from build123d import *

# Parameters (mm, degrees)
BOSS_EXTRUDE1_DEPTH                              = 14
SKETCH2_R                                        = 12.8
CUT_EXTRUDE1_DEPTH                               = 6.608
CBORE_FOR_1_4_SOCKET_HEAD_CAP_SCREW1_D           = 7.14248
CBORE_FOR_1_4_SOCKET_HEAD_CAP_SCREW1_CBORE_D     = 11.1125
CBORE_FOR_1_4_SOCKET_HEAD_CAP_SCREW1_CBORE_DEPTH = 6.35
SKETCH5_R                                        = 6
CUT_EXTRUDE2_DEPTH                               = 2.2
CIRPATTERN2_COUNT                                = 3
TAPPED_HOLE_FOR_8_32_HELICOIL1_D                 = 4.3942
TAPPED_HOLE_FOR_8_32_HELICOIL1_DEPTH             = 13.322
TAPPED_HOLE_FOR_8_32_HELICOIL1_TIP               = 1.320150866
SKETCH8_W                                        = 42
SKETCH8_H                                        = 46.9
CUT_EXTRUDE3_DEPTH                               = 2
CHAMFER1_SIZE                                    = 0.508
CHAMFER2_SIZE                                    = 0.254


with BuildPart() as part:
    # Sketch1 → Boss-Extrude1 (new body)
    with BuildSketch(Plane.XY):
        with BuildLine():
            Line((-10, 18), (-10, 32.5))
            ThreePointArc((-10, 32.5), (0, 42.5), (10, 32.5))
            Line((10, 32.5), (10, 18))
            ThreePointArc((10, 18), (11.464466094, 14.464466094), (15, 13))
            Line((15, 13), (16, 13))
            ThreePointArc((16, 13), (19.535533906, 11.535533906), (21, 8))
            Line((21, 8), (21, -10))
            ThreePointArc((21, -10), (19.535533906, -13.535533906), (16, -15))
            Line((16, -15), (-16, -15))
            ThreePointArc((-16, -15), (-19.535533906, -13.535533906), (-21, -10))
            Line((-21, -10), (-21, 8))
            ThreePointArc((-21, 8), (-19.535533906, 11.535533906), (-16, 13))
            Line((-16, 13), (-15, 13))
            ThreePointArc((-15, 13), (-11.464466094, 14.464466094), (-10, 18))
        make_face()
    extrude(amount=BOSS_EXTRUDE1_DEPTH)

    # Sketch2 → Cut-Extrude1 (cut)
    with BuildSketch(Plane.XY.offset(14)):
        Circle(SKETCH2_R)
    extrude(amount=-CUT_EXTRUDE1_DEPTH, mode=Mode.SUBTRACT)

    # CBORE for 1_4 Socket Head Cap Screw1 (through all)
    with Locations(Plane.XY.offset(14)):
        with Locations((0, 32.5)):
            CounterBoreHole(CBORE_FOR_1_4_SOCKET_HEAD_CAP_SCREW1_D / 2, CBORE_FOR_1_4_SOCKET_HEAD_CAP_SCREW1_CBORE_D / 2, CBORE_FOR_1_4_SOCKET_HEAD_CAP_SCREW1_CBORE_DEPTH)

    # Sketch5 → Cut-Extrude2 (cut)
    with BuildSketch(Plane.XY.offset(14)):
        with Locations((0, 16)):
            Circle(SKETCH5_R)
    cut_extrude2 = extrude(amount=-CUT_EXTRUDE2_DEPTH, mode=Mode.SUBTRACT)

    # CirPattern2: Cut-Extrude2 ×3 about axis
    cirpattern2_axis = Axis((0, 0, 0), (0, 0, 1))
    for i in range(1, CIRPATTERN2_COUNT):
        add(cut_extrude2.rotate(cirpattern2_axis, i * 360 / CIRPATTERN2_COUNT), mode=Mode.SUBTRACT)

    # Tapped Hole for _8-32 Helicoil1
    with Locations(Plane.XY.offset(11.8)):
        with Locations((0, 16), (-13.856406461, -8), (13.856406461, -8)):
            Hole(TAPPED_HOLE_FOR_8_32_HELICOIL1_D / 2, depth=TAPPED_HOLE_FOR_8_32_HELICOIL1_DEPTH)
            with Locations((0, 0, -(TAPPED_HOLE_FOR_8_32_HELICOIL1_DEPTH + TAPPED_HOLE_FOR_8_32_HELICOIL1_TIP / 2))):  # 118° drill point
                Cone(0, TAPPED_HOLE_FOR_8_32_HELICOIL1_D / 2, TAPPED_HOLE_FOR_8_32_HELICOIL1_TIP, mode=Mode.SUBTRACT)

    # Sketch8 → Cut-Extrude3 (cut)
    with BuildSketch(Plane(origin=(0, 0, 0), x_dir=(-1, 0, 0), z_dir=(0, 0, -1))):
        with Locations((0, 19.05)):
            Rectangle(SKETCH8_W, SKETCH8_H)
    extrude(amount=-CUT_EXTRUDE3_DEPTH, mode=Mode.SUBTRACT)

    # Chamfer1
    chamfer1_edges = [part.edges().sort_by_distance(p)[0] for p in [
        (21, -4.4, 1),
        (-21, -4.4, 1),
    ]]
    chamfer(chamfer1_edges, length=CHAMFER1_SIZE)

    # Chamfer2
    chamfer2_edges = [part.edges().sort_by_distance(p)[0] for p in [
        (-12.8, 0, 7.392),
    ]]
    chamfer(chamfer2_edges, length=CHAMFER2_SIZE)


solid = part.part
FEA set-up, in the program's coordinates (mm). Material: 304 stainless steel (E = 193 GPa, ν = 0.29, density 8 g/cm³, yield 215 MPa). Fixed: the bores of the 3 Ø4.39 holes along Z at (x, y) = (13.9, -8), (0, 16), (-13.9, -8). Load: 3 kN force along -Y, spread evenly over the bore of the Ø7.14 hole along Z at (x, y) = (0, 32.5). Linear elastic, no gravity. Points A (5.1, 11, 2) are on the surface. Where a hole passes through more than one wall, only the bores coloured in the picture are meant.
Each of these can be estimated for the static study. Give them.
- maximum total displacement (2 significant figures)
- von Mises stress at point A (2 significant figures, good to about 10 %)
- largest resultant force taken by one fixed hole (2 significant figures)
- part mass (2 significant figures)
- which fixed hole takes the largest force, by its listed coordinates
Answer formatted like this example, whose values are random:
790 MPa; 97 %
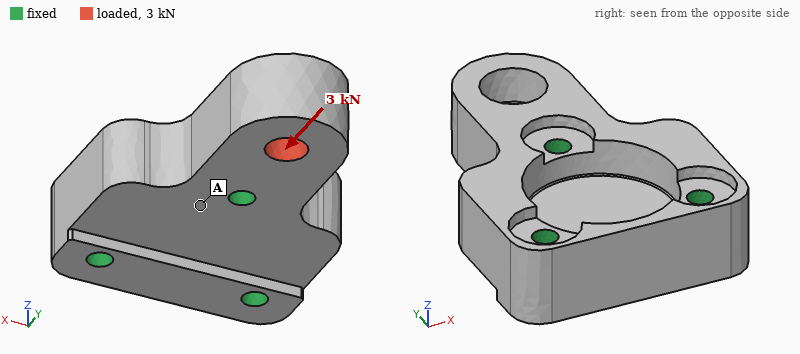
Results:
7.4 µm; 8.3 MPa; 2.4 kN; 130 g; (0, 16)
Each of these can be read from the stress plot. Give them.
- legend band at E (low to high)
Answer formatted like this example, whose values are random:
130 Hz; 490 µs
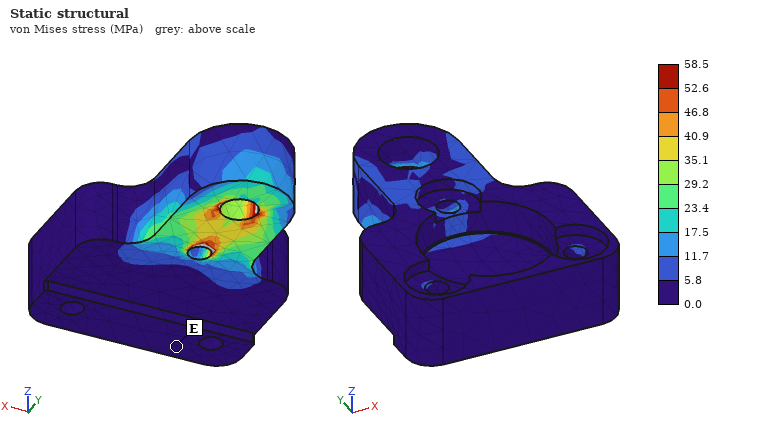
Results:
0.0 to 5.8 MPa
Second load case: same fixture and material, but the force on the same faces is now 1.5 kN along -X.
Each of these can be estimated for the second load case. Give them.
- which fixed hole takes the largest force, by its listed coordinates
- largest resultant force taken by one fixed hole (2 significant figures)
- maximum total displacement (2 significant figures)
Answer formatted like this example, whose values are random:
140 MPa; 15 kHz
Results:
(0, 16); 1.6 kN; 10 µm
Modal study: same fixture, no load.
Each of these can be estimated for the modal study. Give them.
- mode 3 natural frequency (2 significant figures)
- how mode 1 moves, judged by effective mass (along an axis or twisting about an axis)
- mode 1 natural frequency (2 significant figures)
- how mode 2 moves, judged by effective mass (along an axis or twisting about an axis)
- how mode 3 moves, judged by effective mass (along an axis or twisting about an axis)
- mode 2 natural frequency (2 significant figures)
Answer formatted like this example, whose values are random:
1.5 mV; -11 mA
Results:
21 kHz; along Z; 12 kHz; along X; twisting about Y; 14 kHz
